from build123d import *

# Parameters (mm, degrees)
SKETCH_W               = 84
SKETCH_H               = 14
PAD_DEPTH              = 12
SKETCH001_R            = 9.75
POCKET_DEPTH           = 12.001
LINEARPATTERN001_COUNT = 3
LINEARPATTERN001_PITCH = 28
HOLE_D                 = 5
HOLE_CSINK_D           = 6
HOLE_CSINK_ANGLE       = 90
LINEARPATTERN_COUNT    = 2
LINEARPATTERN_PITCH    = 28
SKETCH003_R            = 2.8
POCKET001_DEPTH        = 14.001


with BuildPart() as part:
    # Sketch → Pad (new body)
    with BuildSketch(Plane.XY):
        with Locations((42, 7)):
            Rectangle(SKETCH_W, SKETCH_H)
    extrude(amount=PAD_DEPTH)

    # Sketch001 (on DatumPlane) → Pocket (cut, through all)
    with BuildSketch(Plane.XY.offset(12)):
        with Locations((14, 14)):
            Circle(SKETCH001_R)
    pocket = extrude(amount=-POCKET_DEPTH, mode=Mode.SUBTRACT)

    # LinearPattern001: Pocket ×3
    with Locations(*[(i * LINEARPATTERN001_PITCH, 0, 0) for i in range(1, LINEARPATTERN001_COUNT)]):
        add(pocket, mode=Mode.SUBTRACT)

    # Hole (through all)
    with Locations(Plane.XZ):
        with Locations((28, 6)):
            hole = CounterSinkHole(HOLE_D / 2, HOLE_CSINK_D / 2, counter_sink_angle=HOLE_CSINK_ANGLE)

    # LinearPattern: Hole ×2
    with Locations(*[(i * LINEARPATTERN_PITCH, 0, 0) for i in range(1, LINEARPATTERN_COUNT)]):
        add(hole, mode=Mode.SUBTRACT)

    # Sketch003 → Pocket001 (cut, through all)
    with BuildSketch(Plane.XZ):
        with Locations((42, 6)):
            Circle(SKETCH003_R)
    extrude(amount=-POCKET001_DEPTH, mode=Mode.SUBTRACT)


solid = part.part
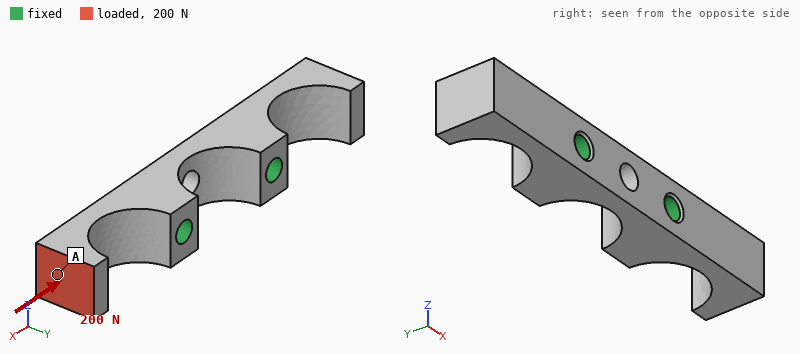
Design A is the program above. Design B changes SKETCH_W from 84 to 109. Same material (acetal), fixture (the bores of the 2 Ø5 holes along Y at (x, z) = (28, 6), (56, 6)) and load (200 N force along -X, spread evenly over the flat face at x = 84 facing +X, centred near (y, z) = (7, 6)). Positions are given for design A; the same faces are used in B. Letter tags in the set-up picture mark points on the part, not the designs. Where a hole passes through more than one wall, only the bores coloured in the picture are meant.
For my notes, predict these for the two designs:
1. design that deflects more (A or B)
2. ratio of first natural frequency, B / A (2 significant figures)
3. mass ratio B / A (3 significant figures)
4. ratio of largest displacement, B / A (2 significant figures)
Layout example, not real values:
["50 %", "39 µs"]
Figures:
["B", "0.40", "1.52", "1.6"]
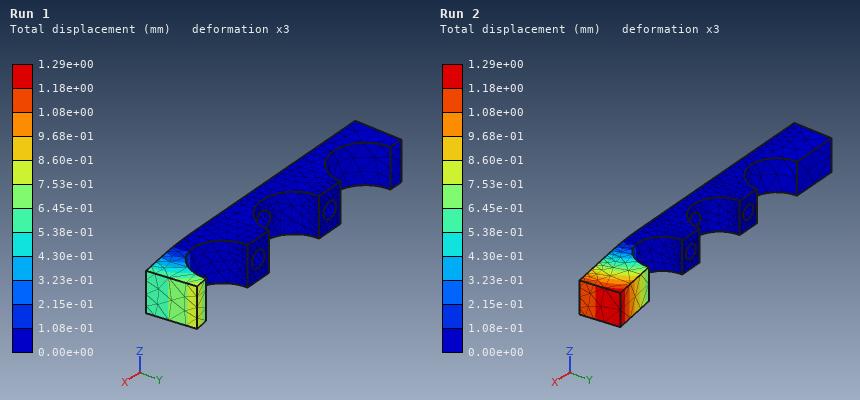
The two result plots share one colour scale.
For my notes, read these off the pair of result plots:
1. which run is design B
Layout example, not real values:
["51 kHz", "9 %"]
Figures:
["Run 2"]
